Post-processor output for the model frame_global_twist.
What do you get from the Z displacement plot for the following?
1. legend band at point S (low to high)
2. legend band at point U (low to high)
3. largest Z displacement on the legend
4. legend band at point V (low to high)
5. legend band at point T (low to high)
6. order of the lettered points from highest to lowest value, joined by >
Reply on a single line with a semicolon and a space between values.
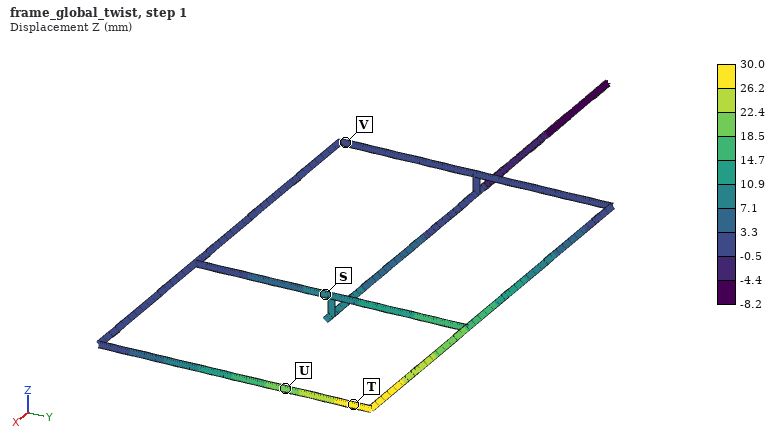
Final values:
7.1 to 10.9 mm; 18.5 to 22.4 mm; 30.0 mm; -0.5 to 3.3 mm; 26.2 to 30.0 mm; T > U > S > V
